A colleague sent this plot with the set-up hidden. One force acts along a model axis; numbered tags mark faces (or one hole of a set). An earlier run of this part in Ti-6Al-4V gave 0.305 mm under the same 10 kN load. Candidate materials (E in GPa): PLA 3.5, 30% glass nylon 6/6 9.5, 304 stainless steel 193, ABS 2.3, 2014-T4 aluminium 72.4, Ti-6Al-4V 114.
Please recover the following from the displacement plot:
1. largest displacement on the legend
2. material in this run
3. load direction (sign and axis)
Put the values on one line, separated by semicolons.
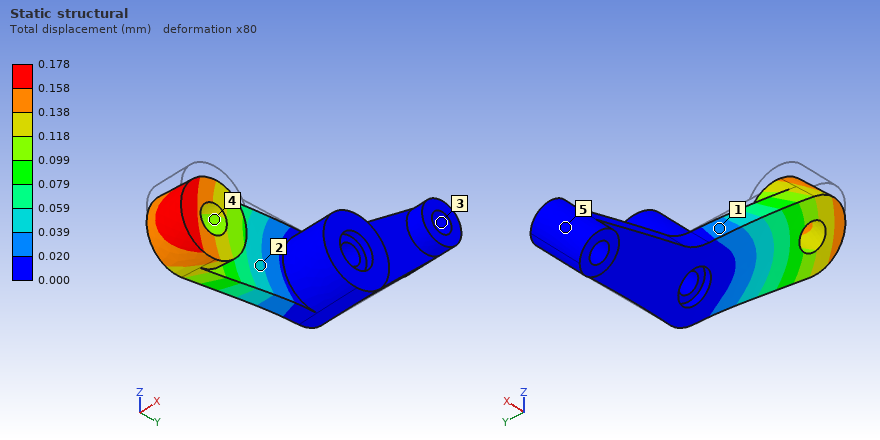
0.178 mm; 304 stainless steel; -Z
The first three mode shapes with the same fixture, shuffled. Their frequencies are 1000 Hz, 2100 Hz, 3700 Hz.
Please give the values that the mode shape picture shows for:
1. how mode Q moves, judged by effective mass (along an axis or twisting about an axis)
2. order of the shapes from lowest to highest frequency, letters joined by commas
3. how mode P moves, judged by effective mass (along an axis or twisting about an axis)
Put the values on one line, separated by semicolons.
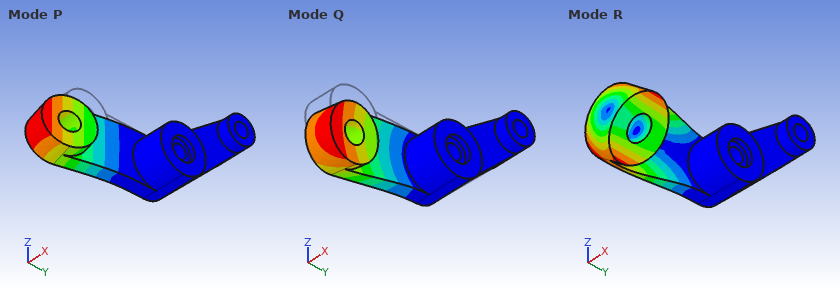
along Z; P, Q, R; along X
